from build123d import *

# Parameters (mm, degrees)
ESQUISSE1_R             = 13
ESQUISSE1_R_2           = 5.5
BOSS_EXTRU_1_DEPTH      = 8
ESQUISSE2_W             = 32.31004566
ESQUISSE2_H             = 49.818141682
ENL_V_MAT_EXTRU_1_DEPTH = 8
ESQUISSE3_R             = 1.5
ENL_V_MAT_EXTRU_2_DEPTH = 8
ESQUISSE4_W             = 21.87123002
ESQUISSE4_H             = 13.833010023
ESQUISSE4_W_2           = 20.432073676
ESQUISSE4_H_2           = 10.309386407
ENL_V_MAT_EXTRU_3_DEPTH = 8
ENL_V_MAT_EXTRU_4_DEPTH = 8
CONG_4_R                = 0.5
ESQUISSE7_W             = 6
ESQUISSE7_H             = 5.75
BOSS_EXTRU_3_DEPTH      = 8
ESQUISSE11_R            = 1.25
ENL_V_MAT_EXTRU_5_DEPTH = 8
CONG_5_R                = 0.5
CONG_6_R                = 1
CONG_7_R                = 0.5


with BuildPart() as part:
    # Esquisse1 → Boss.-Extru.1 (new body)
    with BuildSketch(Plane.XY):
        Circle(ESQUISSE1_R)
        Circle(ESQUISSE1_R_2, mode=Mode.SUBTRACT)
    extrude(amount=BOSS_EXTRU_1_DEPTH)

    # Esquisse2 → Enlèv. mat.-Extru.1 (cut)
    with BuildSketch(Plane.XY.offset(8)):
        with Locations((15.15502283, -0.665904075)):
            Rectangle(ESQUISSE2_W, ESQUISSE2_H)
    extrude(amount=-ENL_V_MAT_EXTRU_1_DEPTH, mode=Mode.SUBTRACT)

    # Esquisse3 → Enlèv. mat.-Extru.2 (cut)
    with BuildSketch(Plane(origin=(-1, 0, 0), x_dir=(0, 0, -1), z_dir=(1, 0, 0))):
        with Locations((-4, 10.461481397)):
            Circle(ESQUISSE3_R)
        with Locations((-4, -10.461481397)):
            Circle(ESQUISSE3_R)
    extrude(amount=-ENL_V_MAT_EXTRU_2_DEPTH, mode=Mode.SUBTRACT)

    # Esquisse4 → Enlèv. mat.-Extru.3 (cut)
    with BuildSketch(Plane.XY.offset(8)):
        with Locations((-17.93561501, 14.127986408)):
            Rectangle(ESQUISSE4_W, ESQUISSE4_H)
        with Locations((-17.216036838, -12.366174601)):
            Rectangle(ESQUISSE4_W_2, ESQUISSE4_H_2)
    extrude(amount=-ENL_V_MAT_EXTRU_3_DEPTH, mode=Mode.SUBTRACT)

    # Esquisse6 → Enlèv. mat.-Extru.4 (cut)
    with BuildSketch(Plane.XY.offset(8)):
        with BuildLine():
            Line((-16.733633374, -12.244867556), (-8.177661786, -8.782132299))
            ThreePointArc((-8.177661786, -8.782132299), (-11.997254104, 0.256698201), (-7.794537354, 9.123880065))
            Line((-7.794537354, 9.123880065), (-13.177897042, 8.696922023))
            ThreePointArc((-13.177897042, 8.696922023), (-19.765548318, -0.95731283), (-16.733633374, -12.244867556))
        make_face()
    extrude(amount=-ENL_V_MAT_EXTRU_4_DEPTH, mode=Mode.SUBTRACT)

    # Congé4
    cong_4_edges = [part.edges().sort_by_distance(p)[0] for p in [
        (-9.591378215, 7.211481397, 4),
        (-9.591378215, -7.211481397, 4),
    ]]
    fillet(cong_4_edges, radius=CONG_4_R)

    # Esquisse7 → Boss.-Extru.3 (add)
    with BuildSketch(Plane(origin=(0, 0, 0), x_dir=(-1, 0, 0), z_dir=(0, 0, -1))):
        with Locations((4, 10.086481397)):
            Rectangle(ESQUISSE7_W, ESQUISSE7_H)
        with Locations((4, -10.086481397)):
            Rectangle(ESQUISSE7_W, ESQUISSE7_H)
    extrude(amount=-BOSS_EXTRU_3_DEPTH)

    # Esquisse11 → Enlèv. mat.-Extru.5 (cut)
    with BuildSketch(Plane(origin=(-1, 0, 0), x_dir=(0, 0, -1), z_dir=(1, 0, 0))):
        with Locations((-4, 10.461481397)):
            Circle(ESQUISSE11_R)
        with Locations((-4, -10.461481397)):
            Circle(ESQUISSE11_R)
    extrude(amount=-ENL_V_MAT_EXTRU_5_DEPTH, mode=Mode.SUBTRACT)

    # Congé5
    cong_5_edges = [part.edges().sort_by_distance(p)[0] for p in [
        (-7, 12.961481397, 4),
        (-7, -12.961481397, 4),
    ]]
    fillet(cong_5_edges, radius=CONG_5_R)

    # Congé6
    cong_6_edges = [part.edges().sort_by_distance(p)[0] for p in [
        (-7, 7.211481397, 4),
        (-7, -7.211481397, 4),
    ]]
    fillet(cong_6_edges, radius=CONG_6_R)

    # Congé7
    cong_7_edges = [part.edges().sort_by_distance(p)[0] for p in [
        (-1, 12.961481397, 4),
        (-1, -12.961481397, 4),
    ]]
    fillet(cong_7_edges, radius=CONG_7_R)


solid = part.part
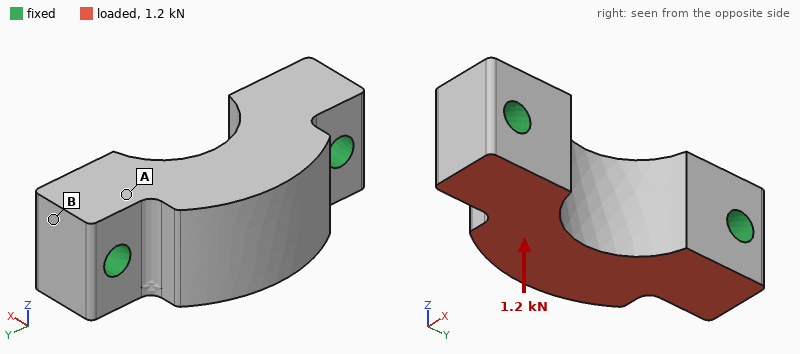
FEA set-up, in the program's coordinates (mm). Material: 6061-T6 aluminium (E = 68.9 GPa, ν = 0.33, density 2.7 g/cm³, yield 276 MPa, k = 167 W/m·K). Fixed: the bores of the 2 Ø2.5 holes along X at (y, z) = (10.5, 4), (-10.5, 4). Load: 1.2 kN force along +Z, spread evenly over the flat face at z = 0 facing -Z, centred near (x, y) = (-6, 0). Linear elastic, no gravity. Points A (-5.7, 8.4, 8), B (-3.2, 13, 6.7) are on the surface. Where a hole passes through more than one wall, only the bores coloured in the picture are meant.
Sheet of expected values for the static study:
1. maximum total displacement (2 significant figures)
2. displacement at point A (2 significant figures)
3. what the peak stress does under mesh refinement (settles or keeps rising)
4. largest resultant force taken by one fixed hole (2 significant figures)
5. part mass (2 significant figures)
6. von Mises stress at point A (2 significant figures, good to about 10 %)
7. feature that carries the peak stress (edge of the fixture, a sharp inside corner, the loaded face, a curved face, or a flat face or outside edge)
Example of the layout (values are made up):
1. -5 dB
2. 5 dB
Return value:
1. 12 µm
2. 3.0 µm
3. keeps rising
4. 600 N
5. 3.7 g
6. 28 MPa
7. edge of the fixture
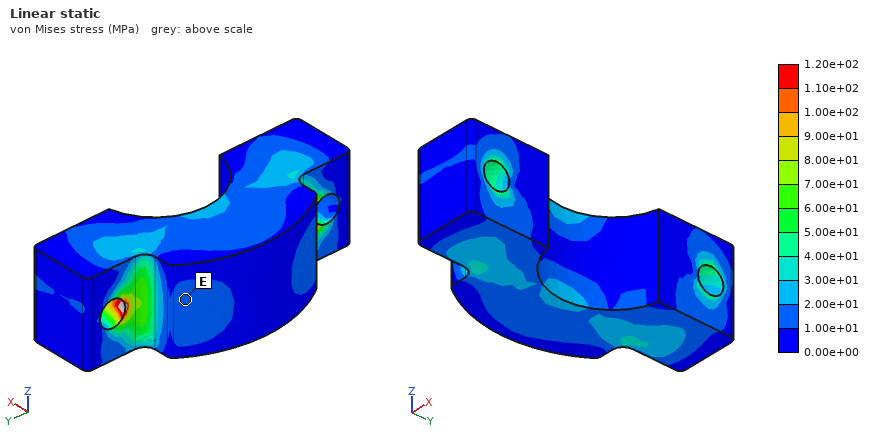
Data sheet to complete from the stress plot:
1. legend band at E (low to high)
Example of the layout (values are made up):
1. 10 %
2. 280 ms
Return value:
1. 1.00e+01 to 2.00e+01 MPa
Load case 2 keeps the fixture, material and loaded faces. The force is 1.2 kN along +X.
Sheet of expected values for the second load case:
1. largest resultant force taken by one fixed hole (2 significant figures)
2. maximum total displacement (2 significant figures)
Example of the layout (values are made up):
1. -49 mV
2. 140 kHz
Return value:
1. 640 N
2. 13 µm
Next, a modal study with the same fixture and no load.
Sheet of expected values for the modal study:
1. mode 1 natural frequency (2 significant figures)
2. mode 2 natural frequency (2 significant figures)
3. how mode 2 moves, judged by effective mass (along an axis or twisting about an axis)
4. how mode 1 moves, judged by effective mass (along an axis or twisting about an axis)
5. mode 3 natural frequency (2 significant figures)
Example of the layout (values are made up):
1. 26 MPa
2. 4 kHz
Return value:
1. 32 kHz
2. 55 kHz
3. along X
4. along Z
5. 72 kHz
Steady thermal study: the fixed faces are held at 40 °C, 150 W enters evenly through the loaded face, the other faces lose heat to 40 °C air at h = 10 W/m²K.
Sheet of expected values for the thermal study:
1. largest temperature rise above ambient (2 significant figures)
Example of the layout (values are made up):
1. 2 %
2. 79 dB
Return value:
1. 62 K
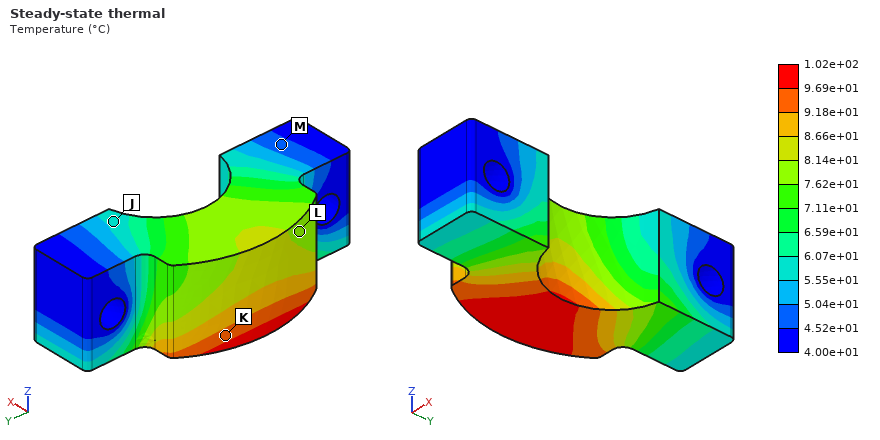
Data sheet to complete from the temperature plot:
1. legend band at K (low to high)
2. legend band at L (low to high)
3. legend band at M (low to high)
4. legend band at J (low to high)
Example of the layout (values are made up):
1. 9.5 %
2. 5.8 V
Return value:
1. 9.18e+01 to 9.69e+01 °C
2. 7.62e+01 to 8.14e+01 °C
3. 4.52e+01 to 5.04e+01 °C
4. 5.55e+01 to 6.07e+01 °C
